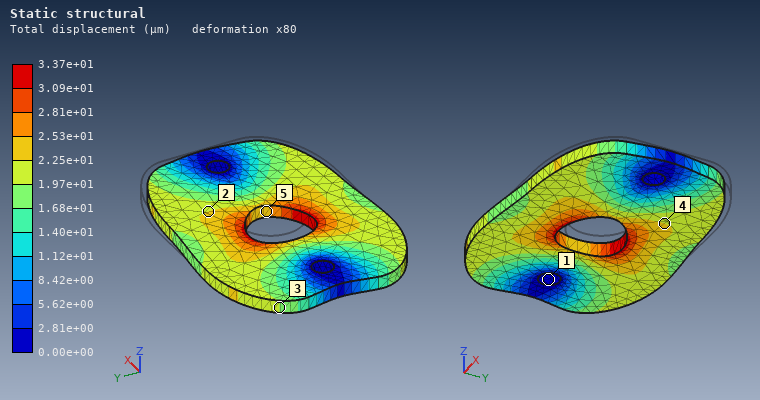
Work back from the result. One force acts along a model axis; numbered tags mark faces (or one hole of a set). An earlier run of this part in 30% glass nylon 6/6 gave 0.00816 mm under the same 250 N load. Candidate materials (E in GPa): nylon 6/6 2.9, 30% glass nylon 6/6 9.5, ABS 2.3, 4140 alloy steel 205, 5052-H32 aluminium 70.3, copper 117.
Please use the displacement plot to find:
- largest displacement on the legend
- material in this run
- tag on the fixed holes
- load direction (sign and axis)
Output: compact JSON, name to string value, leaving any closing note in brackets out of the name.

{"largest displacement on the legend": "3.37e+01 µm", "material in this run": "ABS", "tag on the fixed holes": "1", "load direction": "-X"}
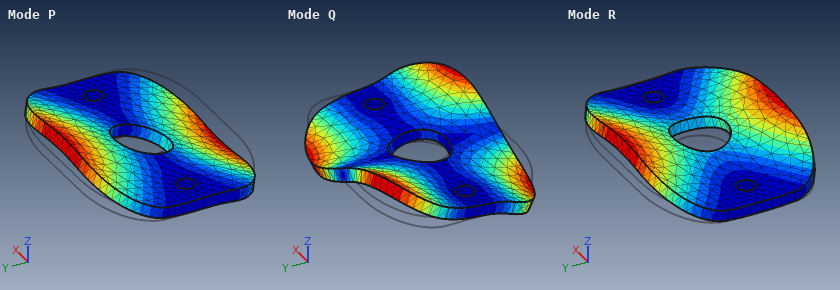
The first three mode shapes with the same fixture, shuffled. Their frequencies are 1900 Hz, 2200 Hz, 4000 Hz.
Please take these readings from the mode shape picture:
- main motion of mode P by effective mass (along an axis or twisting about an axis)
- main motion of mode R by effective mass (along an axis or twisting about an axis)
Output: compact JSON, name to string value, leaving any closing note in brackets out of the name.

{"main motion of mode P by effective mass": "twisting about X", "main motion of mode R by effective mass": "along Z"}
